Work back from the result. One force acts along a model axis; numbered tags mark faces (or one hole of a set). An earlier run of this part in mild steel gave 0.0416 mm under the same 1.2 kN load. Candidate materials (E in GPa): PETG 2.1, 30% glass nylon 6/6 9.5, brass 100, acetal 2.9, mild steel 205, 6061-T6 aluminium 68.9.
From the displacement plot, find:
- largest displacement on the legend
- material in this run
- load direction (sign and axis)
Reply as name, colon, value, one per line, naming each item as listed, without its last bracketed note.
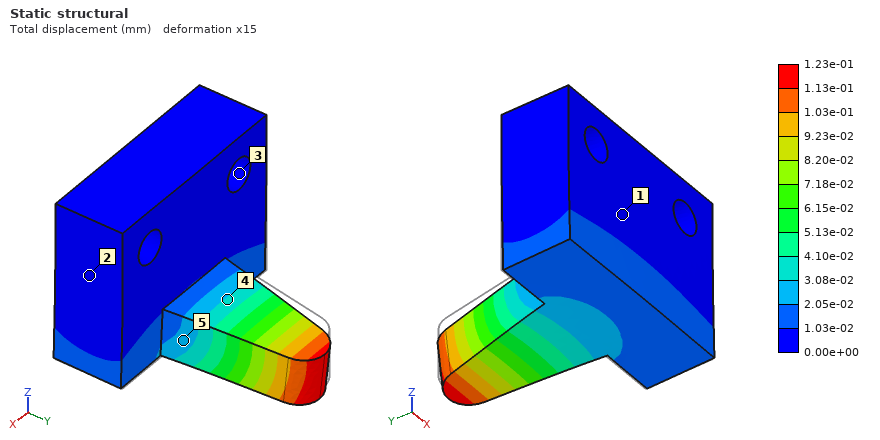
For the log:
largest displacement on the legend: 1.23e-01 mm
material in this run: 6061-T6 aluminium
load direction: -Z
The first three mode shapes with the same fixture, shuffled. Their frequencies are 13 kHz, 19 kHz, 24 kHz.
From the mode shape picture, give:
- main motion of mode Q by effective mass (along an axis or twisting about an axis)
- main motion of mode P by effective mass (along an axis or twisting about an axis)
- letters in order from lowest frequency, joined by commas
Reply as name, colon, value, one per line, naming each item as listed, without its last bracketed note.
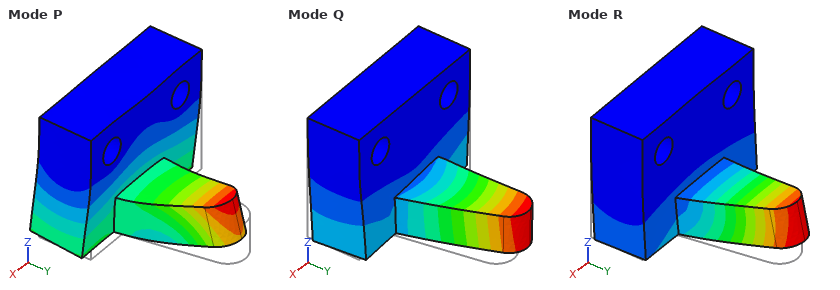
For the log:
main motion of mode Q by effective mass: along X
main motion of mode P by effective mass: along Y
letters in order from lowest frequency, joined by commas: R, Q, P
